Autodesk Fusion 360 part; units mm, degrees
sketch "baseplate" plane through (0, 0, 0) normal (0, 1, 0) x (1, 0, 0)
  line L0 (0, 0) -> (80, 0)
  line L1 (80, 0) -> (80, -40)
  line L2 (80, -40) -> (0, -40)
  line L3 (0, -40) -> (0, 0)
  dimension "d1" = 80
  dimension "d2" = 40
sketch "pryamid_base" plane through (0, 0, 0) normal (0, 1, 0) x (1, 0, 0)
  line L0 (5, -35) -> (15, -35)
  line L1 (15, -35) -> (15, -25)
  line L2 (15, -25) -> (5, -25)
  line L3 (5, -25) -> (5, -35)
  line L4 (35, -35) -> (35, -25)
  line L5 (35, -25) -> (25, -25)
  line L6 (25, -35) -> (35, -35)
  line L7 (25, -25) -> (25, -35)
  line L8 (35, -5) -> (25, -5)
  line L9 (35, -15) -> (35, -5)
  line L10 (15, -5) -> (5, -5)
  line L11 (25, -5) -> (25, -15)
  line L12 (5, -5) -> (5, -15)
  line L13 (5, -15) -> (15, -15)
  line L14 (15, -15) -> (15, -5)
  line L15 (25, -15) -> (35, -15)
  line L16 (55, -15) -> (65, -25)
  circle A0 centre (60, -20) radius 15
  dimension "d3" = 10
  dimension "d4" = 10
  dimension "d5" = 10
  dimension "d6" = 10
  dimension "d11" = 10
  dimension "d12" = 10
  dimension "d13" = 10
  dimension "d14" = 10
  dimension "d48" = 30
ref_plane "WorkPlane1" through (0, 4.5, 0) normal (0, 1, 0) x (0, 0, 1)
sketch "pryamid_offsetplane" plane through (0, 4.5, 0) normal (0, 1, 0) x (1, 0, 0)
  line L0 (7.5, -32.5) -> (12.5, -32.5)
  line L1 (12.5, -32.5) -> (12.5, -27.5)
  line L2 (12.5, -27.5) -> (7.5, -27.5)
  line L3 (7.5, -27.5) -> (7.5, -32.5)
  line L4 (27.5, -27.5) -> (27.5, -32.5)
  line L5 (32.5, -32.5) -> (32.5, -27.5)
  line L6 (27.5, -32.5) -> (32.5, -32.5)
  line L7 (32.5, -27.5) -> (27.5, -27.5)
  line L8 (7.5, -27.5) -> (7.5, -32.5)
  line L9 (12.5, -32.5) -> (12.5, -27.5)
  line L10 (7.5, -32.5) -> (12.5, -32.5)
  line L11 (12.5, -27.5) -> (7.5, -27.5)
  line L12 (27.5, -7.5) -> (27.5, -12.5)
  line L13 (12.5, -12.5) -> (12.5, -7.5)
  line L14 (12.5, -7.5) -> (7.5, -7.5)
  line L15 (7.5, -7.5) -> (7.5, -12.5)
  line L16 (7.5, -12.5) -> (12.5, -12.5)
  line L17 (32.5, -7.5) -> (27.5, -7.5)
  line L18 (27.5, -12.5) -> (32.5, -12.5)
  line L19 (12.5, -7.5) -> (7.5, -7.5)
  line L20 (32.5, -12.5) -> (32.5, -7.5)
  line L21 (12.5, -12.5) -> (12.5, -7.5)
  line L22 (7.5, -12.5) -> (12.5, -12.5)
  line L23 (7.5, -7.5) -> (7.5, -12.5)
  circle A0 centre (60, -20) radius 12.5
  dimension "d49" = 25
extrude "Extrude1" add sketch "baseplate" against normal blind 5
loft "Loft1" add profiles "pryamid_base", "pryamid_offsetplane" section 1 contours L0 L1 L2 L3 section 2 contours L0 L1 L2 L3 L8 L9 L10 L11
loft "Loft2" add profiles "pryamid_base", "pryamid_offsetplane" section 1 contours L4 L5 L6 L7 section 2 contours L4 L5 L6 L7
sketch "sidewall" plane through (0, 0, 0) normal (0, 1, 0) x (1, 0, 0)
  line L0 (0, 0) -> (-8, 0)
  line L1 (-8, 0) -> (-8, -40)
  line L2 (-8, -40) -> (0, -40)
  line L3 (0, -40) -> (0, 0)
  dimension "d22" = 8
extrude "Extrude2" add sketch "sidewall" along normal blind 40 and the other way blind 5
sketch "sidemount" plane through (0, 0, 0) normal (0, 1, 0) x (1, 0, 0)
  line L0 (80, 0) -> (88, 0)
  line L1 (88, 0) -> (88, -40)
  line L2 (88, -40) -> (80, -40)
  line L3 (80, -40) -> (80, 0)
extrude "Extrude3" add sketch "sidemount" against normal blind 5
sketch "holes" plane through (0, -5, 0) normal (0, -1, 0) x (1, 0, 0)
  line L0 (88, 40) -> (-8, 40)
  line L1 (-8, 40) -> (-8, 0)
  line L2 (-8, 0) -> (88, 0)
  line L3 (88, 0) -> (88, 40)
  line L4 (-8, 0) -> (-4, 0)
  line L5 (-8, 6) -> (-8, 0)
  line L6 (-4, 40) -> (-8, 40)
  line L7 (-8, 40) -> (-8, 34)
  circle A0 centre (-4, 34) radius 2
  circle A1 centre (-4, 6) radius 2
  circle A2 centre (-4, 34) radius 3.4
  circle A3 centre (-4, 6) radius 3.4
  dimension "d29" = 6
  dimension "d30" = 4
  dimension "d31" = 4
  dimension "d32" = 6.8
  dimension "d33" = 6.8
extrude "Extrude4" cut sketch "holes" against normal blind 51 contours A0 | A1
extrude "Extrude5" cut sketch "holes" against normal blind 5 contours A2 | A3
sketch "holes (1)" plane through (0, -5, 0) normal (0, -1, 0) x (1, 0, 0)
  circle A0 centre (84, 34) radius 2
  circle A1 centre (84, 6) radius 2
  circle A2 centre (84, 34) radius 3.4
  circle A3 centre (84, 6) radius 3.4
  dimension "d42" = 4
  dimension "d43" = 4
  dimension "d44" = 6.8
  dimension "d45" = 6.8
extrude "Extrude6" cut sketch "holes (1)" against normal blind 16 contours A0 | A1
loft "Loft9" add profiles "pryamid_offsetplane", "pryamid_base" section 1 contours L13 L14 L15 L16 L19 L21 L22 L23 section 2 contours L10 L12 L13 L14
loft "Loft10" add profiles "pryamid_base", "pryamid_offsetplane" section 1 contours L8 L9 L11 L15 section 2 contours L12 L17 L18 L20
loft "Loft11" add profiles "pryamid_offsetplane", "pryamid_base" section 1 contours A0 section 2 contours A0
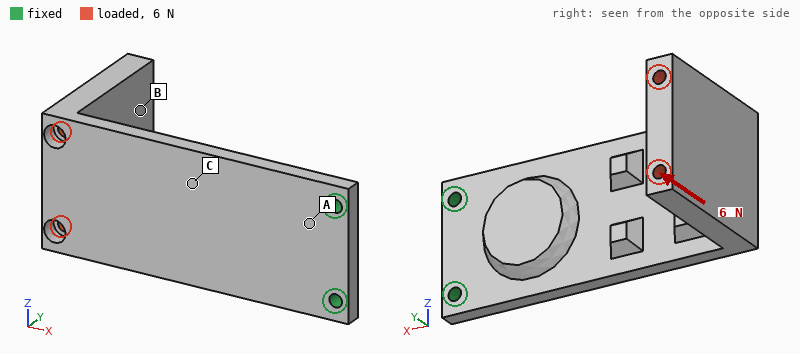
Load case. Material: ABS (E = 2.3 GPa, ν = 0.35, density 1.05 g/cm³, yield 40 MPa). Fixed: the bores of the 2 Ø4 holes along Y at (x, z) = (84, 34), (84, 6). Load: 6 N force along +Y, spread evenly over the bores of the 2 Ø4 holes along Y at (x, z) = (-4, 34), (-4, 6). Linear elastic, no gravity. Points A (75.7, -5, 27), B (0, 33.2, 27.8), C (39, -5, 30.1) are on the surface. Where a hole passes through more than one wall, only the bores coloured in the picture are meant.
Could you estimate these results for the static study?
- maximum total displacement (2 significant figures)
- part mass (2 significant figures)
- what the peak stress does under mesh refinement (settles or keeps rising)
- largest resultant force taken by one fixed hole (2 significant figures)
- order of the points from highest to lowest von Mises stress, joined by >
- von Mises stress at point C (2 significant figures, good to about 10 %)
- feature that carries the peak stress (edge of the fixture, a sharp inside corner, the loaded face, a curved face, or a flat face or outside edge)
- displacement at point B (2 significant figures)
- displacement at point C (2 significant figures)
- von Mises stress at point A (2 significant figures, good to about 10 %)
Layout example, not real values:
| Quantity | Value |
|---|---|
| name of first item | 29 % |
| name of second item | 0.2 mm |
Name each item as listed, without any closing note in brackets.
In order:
| Quantity | Value |
|---|---|
| maximum total displacement | 1.3 mm |
| part mass | 36 g |
| what the peak stress does under mesh refinement | keeps rising |
| largest resultant force taken by one fixed hole | 4.6 N |
| order of the points from highest to lowest von Mises stress, joined by > | A > C > B |
| von Mises stress at point C | 1.4 MPa |
| feature that carries the peak stress | edge of the fixture |
| displacement at point B | 1.1 mm |
| displacement at point C | 0.34 mm |
| von Mises stress at point A | 2.4 MPa |
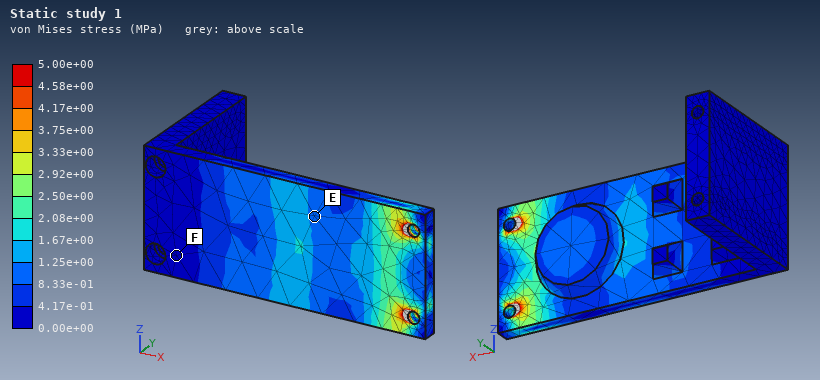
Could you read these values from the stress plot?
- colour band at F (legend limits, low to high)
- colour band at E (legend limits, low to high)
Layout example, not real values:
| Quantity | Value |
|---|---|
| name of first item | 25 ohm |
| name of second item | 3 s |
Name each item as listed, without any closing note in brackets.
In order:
| Quantity | Value |
|---|---|
| colour band at F | 0.00e+00 to 4.17e-01 MPa |
| colour band at E | 8.33e-01 to 1.25e+00 MPa |
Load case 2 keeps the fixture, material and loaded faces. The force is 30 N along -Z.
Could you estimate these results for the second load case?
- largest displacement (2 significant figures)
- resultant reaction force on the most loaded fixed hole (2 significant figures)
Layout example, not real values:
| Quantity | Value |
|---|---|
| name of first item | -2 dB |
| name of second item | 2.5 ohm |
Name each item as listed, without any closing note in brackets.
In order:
| Quantity | Value |
|---|---|
| largest displacement | 1.1 mm |
| resultant reaction force on the most loaded fixed hole | 94 N |
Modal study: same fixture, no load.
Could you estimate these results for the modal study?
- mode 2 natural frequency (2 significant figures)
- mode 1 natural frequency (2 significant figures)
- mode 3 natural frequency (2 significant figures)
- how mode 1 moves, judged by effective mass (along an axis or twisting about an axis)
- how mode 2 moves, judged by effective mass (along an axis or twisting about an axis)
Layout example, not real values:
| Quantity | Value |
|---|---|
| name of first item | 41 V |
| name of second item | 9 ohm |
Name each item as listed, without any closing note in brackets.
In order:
| Quantity | Value |
|---|---|
| mode 2 natural frequency | 260 Hz |
| mode 1 natural frequency | 87 Hz |
| mode 3 natural frequency | 360 Hz |
| how mode 1 moves, judged by effective mass | along Y |
| how mode 2 moves, judged by effective mass | along Z |
